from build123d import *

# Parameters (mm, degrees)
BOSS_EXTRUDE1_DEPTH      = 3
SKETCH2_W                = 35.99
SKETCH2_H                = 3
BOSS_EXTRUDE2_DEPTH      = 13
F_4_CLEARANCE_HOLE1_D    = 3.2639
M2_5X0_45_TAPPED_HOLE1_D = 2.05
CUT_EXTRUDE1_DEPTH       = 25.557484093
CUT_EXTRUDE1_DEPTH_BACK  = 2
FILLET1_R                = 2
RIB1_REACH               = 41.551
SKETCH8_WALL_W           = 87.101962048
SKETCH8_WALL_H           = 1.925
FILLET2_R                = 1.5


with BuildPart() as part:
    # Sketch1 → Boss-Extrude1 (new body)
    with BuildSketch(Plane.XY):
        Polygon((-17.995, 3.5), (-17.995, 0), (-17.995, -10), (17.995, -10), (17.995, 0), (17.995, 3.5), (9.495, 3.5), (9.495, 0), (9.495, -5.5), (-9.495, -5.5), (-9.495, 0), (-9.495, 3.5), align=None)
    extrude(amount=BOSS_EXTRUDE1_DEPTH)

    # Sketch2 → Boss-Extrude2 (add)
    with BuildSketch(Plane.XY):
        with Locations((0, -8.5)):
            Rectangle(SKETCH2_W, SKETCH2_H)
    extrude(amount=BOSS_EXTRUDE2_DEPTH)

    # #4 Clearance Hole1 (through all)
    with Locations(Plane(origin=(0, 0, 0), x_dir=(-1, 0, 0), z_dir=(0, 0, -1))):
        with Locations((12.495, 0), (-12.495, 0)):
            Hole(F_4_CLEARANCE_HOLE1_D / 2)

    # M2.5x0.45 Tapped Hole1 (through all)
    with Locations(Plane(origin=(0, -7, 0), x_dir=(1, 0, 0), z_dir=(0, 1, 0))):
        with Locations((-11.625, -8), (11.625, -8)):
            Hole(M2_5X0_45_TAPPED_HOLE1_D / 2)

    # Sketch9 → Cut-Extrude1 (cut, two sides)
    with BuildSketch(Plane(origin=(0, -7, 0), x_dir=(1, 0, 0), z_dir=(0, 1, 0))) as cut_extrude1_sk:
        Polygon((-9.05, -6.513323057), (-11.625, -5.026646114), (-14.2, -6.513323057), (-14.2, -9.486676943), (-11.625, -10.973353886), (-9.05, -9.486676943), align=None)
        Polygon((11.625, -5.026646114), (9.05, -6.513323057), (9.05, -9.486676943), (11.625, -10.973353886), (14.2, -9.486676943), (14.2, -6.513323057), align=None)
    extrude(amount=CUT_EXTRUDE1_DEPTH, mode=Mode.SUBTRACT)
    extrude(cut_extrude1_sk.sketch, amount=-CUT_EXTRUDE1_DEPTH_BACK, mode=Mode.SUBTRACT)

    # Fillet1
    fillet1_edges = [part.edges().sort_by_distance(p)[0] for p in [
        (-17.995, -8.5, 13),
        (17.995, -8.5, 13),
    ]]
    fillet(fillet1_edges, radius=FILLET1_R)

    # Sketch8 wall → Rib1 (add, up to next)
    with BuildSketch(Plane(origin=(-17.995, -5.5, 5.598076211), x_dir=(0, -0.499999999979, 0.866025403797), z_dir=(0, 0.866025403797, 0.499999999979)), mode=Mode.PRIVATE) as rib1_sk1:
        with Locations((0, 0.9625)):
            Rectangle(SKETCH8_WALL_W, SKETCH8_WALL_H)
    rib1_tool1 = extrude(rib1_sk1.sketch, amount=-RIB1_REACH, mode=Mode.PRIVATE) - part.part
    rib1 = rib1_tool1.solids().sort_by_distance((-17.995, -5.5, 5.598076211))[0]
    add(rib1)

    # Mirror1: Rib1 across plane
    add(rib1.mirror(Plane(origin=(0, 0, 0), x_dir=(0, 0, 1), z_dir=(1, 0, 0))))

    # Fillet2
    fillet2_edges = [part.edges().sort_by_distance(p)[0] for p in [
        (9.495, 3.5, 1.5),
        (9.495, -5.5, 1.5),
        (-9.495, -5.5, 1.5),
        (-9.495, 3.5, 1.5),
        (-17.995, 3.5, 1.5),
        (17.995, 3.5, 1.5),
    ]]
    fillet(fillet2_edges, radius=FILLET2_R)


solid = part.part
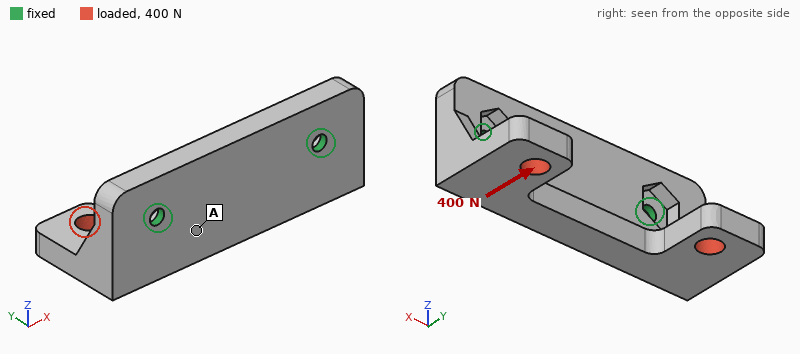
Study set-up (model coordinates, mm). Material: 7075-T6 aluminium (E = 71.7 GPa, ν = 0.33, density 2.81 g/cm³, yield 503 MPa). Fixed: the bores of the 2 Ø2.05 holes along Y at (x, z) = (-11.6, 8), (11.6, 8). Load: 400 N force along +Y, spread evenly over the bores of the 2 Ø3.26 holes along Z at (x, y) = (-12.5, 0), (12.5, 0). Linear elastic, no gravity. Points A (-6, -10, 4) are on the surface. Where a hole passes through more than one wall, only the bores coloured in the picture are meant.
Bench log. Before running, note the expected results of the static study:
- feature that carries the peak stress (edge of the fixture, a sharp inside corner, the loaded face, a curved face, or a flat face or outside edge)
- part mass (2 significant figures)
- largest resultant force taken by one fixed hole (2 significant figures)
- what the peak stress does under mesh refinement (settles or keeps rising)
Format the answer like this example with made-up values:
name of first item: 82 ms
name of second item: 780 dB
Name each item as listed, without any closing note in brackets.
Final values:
feature that carries the peak stress: edge of the fixture
part mass: 5.3 g
largest resultant force taken by one fixed hole: 200 N
what the peak stress does under mesh refinement: keeps rising
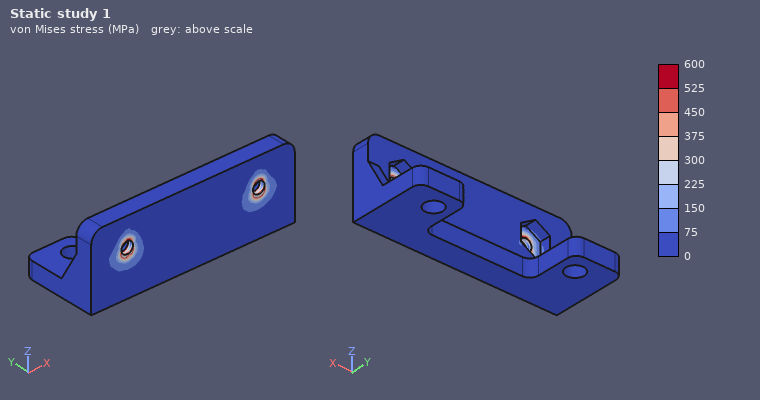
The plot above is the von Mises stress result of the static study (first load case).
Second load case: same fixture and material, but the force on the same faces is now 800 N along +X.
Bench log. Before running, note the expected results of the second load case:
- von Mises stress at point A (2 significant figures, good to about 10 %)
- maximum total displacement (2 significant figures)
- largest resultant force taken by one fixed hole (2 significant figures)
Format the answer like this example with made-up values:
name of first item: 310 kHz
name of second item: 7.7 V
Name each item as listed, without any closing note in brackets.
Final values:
von Mises stress at point A: 62 MPa
maximum total displacement: 0.12 mm
largest resultant force taken by one fixed hole: 550 N
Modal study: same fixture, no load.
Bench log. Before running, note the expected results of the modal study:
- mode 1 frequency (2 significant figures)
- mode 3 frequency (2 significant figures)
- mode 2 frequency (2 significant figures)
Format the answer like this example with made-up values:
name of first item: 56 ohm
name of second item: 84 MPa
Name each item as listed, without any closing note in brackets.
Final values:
mode 1 frequency: 4800 Hz
mode 3 frequency: 12 kHz
mode 2 frequency: 8200 Hz
